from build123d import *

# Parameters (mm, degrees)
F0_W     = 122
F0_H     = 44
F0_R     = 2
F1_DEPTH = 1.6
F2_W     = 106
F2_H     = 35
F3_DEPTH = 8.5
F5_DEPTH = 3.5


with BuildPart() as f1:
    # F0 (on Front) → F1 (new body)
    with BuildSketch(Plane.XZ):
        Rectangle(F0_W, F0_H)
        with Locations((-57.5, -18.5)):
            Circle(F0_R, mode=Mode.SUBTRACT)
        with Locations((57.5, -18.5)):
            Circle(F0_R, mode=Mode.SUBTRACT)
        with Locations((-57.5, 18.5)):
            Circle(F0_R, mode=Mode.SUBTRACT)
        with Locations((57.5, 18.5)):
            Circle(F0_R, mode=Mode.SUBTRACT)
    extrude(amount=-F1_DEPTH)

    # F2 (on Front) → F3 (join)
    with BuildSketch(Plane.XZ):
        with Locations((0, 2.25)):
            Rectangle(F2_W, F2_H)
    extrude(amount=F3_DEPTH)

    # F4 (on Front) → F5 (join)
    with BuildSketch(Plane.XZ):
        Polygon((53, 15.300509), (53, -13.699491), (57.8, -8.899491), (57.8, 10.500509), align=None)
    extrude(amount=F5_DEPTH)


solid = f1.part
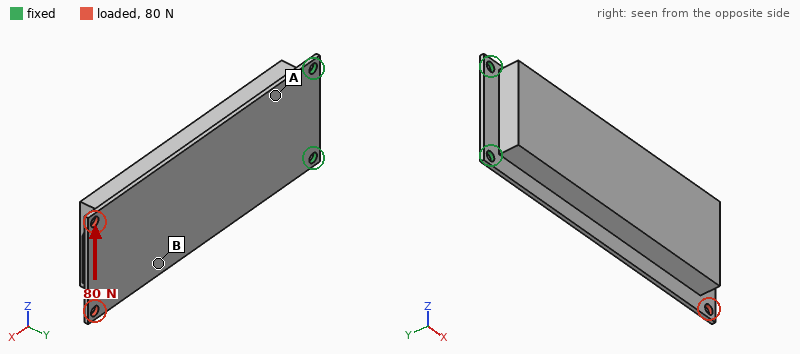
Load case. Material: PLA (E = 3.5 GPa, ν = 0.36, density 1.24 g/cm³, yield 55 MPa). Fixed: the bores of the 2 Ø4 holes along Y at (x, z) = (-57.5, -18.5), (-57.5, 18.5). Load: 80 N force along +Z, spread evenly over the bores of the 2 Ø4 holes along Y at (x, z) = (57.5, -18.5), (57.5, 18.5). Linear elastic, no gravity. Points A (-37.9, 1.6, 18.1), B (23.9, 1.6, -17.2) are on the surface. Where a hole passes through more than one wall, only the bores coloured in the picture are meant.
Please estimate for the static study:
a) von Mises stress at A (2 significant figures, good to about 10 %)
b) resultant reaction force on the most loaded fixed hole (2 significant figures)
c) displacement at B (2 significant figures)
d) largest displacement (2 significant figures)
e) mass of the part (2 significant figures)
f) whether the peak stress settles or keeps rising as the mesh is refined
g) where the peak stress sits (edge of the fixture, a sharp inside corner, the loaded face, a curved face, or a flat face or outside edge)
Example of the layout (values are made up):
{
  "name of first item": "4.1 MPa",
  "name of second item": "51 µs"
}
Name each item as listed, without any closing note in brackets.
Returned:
{
  "von Mises stress at A": "5.0 MPa",
  "resultant reaction force on the most loaded fixed hole": "250 N",
  "displacement at B": "0.44 mm",
  "largest displacement": "0.71 mm",
  "mass of the part": "50 g",
  "whether the peak stress settles or keeps rising as the mesh is refined": "keeps rising",
  "where the peak stress sits": "edge of the fixture"
}
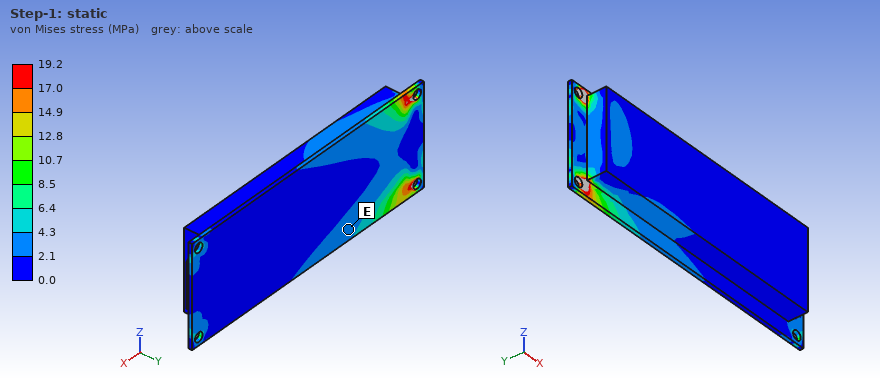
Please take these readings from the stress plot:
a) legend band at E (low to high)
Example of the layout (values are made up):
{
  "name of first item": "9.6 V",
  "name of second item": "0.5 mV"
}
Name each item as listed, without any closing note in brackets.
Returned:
{
  "legend band at E": "2.1 to 4.3 MPa"
}
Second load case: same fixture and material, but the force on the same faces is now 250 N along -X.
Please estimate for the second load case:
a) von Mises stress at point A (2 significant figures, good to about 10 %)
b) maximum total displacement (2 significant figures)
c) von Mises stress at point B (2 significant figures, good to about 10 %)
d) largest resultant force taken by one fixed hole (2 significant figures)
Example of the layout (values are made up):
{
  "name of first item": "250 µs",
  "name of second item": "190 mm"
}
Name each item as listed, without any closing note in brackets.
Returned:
{
  "von Mises stress at point A": "2.5 MPa",
  "maximum total displacement": "0.69 mm",
  "von Mises stress at point B": "2.5 MPa",
  "largest resultant force taken by one fixed hole": "130 N"
}
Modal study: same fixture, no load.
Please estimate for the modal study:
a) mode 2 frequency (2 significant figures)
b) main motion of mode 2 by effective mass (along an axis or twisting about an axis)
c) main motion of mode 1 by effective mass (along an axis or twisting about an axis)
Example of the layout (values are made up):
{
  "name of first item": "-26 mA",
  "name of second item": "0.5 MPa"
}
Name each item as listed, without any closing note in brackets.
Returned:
{
  "mode 2 frequency": "500 Hz",
  "main motion of mode 2 by effective mass": "along Z",
  "main motion of mode 1 by effective mass": "along Y"
}
